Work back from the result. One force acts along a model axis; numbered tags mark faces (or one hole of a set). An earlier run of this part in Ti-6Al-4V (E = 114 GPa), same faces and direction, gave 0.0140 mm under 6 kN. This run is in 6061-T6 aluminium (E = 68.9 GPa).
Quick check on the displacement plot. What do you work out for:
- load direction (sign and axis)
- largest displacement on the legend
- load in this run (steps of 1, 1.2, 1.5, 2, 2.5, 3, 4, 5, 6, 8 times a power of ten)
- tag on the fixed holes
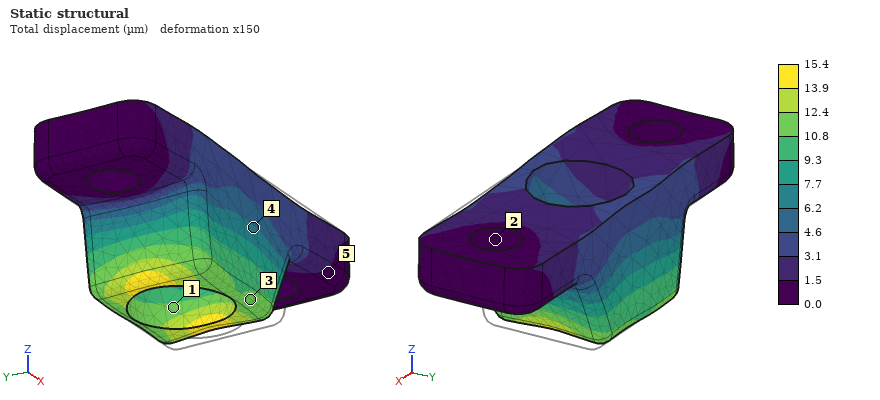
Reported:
-X
15.4 µm
4 kN
2
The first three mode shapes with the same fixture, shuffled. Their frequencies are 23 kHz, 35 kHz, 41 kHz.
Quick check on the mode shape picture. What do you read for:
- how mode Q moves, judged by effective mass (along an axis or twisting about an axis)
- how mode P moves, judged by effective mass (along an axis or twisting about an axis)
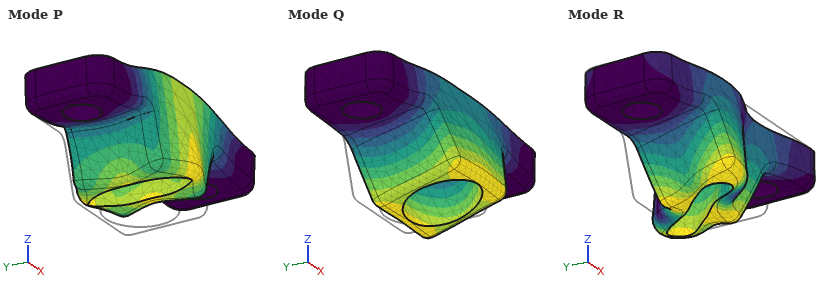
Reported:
along Y
along Z
